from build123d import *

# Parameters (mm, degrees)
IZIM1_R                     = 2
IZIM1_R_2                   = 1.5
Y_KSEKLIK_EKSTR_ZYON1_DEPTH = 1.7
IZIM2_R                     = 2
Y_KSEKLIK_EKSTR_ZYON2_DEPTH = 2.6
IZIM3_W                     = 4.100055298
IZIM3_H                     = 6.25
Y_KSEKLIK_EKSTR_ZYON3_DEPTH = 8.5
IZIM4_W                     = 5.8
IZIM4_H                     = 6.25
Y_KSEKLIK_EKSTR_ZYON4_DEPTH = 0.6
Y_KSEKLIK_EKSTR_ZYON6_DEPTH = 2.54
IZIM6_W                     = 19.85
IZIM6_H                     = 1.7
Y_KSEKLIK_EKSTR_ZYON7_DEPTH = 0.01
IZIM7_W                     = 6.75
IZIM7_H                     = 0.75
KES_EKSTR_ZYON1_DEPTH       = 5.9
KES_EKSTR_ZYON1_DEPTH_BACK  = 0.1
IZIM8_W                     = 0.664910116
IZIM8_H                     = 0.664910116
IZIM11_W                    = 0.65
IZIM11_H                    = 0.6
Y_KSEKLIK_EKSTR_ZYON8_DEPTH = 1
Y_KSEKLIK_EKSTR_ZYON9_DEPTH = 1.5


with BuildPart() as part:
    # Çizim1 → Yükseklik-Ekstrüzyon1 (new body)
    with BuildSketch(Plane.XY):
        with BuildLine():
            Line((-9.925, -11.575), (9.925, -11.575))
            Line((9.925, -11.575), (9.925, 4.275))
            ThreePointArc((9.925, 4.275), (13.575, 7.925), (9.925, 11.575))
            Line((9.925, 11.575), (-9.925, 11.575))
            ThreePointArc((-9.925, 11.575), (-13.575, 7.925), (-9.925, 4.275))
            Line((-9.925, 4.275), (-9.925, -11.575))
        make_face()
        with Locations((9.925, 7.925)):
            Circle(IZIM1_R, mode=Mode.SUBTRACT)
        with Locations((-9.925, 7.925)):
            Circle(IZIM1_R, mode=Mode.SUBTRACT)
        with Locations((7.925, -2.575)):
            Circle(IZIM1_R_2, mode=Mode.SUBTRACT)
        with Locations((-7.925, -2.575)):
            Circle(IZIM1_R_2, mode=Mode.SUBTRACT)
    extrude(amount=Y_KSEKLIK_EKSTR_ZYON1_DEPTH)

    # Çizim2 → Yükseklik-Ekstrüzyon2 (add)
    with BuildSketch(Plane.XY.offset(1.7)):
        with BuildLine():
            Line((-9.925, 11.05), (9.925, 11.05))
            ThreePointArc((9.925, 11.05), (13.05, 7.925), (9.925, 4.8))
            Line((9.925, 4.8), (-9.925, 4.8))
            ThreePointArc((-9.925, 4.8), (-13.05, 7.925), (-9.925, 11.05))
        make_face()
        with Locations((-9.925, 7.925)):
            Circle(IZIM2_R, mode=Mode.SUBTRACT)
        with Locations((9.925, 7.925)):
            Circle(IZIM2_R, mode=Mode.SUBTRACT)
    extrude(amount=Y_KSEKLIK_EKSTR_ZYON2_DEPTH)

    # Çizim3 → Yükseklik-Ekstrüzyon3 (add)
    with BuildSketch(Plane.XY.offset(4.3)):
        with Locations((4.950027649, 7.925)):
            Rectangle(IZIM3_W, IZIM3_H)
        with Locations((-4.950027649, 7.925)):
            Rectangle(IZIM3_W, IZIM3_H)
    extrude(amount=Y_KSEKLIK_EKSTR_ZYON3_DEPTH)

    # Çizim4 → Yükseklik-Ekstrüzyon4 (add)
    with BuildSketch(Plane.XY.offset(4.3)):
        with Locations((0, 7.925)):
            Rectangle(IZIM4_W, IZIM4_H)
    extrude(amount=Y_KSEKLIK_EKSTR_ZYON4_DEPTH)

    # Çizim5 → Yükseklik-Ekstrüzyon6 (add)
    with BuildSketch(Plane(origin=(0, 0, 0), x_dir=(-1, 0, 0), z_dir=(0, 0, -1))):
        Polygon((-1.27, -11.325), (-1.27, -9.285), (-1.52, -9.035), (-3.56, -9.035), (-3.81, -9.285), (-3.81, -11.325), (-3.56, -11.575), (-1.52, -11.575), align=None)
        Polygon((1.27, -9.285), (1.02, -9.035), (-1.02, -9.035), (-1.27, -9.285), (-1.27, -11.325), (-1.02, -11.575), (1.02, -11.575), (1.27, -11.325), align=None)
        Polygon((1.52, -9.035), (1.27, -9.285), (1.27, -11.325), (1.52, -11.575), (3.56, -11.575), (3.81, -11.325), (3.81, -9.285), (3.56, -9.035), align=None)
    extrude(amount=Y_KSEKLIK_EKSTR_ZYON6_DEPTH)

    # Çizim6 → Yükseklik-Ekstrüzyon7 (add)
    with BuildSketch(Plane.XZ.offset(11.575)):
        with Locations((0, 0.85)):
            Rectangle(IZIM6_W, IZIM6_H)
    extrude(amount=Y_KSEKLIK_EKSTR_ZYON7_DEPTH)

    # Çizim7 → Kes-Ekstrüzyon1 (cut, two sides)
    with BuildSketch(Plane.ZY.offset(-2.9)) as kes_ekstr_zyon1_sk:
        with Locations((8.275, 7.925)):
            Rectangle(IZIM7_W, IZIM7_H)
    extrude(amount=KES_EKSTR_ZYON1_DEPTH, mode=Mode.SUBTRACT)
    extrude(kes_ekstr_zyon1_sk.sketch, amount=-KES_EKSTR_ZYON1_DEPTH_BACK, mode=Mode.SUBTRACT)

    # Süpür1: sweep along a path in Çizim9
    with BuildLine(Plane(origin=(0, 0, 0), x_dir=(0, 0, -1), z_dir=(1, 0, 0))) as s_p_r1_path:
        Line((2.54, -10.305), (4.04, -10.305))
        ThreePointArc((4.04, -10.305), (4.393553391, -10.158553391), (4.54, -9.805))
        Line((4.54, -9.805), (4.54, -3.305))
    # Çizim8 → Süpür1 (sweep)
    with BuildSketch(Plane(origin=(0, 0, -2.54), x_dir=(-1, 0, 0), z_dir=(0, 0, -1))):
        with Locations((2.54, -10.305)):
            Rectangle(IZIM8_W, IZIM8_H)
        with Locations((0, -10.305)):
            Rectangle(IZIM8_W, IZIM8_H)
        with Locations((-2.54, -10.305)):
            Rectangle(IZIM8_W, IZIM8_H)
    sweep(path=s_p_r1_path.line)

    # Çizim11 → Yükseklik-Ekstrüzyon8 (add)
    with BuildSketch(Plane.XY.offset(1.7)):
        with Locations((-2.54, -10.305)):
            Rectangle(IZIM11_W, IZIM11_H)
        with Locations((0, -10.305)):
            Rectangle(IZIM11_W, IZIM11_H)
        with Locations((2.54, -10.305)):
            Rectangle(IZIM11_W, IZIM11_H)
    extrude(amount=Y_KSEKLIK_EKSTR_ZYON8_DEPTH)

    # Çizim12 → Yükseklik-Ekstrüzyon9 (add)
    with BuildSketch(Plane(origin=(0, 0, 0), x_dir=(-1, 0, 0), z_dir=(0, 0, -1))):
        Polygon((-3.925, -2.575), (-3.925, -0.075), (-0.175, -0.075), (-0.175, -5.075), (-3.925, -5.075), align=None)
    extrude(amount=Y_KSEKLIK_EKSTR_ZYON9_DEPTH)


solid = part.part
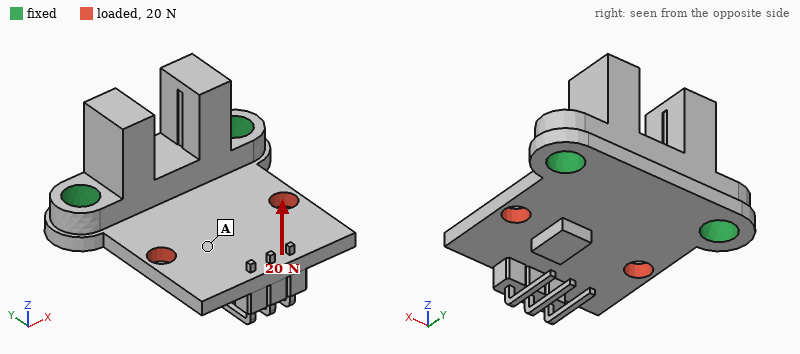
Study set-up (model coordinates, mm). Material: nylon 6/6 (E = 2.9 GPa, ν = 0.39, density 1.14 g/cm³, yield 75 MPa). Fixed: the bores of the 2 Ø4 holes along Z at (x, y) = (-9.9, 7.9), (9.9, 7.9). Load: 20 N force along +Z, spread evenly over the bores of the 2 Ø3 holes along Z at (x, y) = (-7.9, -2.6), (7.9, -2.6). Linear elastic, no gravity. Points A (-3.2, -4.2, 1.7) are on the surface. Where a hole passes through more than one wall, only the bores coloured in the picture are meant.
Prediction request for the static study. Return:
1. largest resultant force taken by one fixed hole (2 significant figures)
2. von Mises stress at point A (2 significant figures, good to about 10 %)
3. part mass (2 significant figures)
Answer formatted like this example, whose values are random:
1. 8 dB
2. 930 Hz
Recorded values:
1. 10 N
2. 1.7 MPa
3. 1.9 g
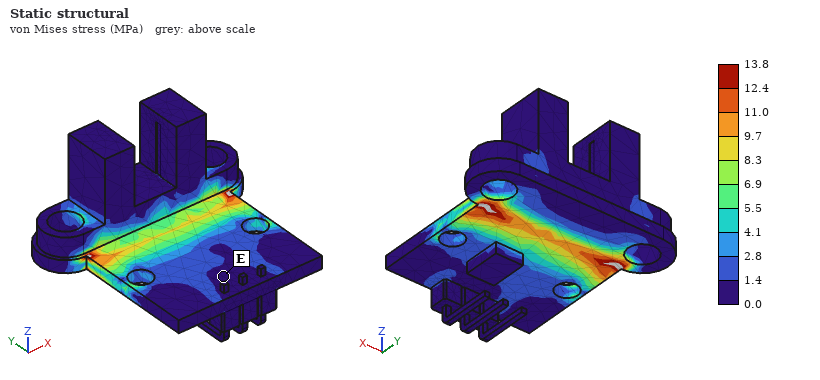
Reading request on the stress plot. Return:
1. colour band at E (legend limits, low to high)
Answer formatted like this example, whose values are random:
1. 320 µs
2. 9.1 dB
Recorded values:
1. 0.0 to 1.4 MPa
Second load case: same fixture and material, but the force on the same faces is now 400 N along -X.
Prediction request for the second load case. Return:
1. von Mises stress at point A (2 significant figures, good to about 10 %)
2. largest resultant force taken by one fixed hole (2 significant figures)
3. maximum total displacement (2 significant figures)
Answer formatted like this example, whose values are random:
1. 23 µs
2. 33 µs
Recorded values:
1. 14 MPa
2. 290 N
3. 0.23 mm
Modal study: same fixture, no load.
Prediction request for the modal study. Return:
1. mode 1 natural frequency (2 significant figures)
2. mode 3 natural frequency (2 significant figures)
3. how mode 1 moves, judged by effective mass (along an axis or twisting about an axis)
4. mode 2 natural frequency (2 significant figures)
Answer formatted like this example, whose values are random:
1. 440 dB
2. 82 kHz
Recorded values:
1. 1300 Hz
2. 2100 Hz
3. along Z
4. 2100 Hz
